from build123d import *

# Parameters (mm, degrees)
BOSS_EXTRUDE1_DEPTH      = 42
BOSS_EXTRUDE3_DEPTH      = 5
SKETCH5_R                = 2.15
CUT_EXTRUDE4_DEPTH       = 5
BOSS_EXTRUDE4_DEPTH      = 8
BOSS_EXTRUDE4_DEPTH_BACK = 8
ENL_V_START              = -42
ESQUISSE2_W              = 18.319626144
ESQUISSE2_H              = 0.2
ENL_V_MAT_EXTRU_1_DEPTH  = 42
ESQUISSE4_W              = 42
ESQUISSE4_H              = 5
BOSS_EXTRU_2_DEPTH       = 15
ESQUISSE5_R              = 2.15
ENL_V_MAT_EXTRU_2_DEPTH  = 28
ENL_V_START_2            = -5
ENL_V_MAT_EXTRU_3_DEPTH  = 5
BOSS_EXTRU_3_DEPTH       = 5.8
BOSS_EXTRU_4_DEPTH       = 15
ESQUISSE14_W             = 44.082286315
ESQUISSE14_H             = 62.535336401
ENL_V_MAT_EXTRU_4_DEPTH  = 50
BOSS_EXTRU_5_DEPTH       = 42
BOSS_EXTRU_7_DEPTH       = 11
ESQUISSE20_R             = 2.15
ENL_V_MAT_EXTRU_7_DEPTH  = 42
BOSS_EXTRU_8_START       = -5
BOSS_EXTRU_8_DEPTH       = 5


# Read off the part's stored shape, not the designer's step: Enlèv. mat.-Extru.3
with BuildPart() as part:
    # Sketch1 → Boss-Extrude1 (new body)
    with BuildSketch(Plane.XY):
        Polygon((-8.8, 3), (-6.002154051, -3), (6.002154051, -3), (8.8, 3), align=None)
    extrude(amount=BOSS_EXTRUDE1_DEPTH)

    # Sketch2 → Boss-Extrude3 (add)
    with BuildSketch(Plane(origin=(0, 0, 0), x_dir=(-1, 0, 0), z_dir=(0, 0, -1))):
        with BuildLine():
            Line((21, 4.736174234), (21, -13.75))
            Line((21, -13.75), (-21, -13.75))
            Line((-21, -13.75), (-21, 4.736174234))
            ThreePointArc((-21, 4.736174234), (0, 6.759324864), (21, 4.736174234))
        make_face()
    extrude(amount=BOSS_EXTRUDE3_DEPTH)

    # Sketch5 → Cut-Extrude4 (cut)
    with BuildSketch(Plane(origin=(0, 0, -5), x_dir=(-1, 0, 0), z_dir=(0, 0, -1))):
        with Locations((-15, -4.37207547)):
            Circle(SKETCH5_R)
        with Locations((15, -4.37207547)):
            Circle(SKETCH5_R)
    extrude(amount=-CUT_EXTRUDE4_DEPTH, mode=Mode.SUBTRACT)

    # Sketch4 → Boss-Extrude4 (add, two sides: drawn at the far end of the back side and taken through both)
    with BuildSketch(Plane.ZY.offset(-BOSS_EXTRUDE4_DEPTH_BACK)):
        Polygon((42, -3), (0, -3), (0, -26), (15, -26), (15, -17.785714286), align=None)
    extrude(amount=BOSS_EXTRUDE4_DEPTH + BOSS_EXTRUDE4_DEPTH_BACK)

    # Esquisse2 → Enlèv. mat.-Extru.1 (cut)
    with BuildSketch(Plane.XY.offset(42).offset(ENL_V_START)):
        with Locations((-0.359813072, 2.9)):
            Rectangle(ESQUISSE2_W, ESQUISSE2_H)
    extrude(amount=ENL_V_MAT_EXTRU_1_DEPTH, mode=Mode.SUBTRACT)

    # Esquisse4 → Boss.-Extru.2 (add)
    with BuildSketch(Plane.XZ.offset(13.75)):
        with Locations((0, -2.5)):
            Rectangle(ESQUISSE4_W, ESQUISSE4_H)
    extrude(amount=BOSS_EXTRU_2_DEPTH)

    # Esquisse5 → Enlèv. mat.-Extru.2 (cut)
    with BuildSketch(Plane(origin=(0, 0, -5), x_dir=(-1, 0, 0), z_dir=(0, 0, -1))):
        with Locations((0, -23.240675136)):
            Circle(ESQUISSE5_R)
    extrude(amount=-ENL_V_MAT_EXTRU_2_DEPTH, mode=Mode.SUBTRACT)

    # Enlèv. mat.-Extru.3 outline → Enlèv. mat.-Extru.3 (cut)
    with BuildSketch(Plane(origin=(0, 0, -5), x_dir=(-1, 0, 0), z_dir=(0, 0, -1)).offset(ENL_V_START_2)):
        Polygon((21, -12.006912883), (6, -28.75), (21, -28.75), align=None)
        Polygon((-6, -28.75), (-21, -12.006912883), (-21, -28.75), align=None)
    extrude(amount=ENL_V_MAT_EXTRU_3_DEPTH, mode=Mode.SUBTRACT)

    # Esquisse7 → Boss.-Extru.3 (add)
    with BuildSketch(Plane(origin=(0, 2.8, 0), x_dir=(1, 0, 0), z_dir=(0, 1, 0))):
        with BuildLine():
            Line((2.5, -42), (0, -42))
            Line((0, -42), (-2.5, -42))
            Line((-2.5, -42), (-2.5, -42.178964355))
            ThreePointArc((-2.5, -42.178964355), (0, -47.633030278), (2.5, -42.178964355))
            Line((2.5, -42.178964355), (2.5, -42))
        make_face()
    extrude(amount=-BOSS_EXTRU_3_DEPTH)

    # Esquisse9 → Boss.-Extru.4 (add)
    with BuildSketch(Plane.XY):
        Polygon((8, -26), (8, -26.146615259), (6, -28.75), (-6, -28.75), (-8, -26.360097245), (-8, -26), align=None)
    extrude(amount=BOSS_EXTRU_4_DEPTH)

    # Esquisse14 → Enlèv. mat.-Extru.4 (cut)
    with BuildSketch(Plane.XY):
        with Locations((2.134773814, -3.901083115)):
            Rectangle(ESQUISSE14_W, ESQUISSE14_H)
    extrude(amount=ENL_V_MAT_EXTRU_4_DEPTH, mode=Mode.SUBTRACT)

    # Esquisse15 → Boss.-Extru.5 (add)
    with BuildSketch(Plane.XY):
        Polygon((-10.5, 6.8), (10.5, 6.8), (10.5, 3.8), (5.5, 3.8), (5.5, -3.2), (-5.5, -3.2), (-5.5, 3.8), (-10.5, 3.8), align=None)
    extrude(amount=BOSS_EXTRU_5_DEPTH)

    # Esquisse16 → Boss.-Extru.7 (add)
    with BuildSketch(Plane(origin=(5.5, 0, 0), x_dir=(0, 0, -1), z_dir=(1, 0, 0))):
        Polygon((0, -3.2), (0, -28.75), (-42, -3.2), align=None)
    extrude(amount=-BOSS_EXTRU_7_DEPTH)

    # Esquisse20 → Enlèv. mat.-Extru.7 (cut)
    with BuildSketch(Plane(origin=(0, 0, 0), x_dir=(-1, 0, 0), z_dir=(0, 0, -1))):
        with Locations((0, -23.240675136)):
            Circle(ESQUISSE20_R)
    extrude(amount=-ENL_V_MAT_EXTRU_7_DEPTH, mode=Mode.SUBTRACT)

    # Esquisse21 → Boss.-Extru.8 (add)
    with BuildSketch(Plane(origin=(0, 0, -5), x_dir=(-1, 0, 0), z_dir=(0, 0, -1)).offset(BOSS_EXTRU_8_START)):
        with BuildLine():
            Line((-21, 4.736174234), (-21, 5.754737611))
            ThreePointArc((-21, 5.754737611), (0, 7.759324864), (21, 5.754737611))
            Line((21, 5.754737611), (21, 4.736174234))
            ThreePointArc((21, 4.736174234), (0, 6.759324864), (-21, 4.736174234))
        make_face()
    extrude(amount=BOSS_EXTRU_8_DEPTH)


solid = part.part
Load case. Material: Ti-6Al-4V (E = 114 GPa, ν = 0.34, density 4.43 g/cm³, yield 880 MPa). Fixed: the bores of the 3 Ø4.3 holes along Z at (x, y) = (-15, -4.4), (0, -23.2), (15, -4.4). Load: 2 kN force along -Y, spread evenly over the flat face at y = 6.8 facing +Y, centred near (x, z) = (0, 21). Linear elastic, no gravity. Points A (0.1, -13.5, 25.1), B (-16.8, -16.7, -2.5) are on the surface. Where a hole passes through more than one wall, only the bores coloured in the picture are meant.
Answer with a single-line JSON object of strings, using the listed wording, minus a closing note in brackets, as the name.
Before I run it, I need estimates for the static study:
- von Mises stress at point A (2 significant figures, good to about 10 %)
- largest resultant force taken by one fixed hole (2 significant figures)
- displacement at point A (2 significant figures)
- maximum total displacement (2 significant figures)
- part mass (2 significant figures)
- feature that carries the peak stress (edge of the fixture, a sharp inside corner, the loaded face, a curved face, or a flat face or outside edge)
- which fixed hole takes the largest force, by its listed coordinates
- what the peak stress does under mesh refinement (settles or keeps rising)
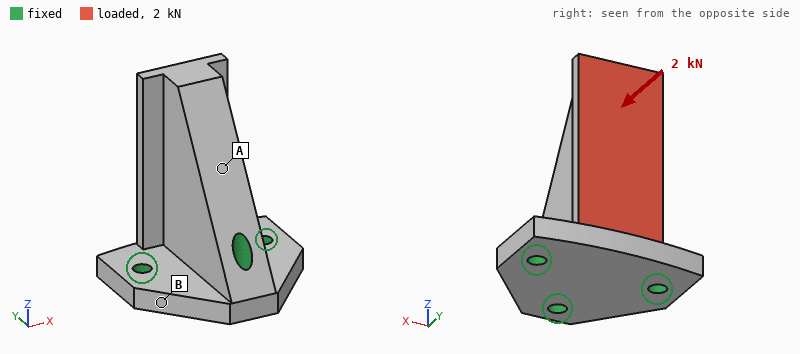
{"von Mises stress at point A": "12 MPa", "largest resultant force taken by one fixed hole": "2.5 kN", "displacement at point A": "8.8 µm", "maximum total displacement": "21 µm", "part mass": "78 g", "feature that carries the peak stress": "edge of the fixture", "which fixed hole takes the largest force, by its listed coordinates": "(0, -23.2)", "what the peak stress does under mesh refinement": "keeps rising"}
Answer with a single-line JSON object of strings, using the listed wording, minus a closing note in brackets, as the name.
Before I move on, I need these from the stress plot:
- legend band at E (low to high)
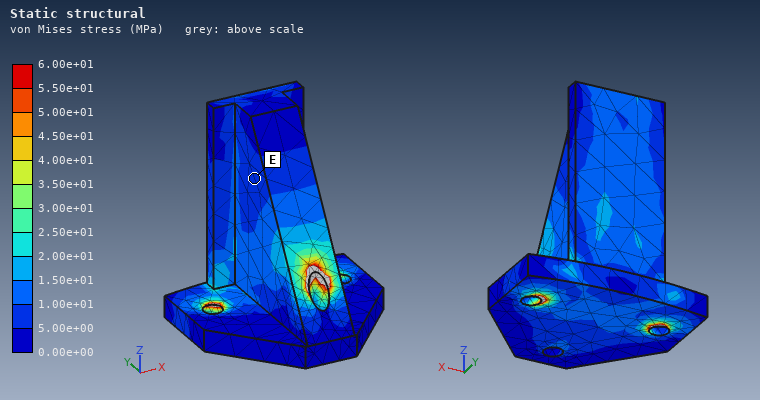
{"legend band at E": "5.00e+00 to 1.00e+01 MPa"}
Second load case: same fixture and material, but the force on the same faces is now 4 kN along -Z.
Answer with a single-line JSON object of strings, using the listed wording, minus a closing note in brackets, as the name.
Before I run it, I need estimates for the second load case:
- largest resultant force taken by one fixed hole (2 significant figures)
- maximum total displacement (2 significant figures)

{"largest resultant force taken by one fixed hole": "2.2 kN", "maximum total displacement": "47 µm"}
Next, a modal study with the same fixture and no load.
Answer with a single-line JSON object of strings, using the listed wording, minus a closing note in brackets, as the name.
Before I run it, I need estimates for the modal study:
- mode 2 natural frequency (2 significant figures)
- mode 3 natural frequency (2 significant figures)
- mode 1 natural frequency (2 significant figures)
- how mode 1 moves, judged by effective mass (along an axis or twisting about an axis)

{"mode 2 natural frequency": "9000 Hz", "mode 3 natural frequency": "19 kHz", "mode 1 natural frequency": "5600 Hz", "how mode 1 moves, judged by effective mass": "along X"}
